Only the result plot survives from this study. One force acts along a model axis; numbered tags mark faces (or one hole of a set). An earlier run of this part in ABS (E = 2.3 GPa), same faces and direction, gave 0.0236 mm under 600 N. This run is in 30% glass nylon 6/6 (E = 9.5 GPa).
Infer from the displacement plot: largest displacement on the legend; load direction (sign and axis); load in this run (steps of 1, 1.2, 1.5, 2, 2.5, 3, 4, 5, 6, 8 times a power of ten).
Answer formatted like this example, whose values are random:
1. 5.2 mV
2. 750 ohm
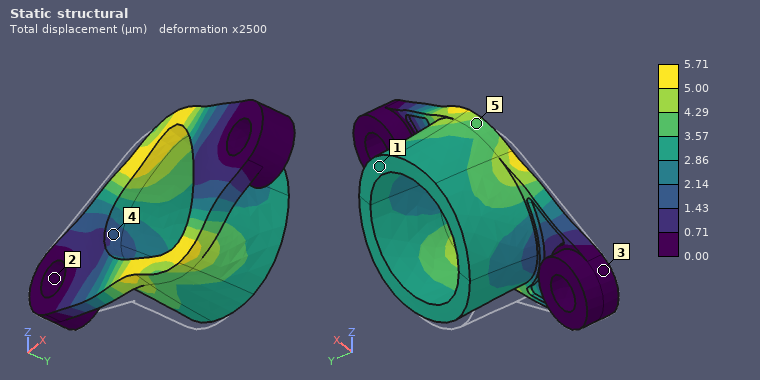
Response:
1. 5.71 µm
2. +X
3. 600 N
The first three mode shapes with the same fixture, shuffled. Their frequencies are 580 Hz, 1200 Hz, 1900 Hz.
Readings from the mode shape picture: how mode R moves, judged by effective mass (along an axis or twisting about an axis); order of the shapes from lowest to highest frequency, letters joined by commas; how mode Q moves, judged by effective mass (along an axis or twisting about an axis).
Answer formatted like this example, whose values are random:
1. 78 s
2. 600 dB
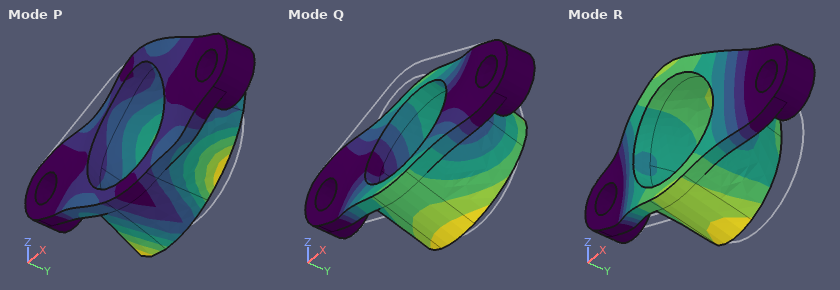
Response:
1. along Y
2. Q, R, P
3. along Z
